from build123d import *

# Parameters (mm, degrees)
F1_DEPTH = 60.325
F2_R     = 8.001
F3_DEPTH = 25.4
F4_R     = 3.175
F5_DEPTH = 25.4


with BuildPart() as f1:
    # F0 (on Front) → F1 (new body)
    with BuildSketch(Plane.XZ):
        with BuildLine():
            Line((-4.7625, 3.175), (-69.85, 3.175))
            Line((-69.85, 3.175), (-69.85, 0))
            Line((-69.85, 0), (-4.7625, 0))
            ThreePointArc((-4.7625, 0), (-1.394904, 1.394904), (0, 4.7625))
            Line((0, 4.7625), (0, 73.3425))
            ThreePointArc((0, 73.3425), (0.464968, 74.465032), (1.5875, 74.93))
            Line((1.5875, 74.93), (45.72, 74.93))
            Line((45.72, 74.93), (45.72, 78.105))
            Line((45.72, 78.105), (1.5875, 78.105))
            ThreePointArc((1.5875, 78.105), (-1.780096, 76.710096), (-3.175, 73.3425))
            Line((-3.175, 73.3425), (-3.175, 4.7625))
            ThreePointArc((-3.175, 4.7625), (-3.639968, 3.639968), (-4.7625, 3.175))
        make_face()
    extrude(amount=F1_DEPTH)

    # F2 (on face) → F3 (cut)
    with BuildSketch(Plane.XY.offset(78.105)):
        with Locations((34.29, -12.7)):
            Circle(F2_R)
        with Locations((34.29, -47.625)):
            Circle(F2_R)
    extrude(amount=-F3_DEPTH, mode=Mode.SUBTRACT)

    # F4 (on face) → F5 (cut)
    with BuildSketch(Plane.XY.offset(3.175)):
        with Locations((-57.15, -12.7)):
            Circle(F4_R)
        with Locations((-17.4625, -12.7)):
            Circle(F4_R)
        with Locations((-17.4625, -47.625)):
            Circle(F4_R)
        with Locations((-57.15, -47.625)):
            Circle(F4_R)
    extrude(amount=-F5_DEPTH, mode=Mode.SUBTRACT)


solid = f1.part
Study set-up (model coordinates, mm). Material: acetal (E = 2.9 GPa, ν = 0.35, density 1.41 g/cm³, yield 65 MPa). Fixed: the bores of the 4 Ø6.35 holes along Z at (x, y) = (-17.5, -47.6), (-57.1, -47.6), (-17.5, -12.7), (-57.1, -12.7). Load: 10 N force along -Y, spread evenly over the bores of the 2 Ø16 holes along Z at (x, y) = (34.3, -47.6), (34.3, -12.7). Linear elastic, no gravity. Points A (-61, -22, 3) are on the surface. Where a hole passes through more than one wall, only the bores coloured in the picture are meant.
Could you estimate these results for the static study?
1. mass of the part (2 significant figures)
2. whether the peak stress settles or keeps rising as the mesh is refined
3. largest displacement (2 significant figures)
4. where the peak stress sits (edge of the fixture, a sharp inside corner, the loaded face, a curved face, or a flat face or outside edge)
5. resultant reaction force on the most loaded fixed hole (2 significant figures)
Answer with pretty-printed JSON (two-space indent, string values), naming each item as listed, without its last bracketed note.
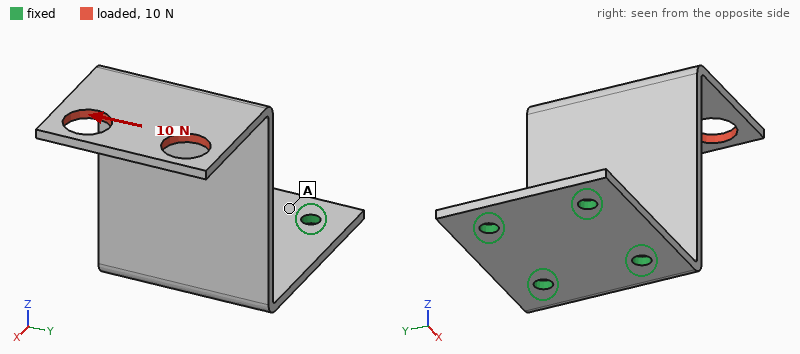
{
  "mass of the part": "48 g",
  "whether the peak stress settles or keeps rising as the mesh is refined": "keeps rising",
  "largest displacement": "1.7 mm",
  "where the peak stress sits": "edge of the fixture",
  "resultant reaction force on the most loaded fixed hole": "23 N"
}
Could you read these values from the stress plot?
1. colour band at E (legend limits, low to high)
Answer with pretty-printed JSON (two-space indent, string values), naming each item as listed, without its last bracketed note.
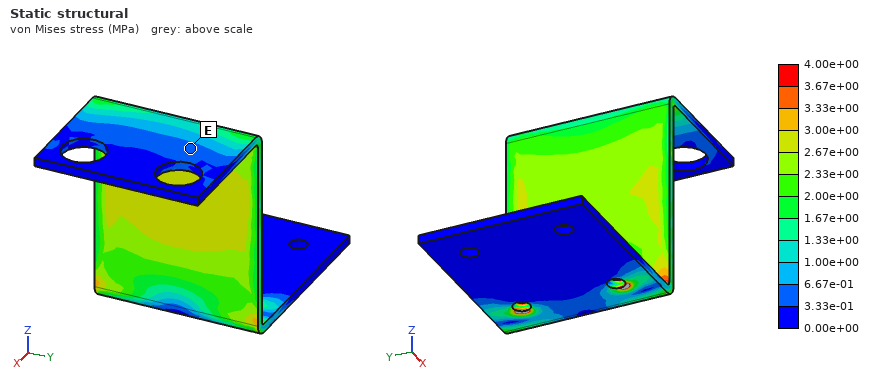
{
  "colour band at E": "3.33e-01 to 6.67e-01 MPa"
}
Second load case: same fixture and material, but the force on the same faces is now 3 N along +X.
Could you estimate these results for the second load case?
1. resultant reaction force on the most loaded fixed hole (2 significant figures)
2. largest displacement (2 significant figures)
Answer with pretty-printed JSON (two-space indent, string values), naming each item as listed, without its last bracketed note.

{
  "resultant reaction force on the most loaded fixed hole": "1.6 N",
  "largest displacement": "1.7 mm"
}
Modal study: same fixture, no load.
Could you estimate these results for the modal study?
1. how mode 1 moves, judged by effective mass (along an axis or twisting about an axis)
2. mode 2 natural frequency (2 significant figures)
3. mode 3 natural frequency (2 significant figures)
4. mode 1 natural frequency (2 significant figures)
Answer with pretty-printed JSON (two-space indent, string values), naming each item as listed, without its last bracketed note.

{
  "how mode 1 moves, judged by effective mass": "along X",
  "mode 2 natural frequency": "160 Hz",
  "mode 3 natural frequency": "240 Hz",
  "mode 1 natural frequency": "56 Hz"
}
